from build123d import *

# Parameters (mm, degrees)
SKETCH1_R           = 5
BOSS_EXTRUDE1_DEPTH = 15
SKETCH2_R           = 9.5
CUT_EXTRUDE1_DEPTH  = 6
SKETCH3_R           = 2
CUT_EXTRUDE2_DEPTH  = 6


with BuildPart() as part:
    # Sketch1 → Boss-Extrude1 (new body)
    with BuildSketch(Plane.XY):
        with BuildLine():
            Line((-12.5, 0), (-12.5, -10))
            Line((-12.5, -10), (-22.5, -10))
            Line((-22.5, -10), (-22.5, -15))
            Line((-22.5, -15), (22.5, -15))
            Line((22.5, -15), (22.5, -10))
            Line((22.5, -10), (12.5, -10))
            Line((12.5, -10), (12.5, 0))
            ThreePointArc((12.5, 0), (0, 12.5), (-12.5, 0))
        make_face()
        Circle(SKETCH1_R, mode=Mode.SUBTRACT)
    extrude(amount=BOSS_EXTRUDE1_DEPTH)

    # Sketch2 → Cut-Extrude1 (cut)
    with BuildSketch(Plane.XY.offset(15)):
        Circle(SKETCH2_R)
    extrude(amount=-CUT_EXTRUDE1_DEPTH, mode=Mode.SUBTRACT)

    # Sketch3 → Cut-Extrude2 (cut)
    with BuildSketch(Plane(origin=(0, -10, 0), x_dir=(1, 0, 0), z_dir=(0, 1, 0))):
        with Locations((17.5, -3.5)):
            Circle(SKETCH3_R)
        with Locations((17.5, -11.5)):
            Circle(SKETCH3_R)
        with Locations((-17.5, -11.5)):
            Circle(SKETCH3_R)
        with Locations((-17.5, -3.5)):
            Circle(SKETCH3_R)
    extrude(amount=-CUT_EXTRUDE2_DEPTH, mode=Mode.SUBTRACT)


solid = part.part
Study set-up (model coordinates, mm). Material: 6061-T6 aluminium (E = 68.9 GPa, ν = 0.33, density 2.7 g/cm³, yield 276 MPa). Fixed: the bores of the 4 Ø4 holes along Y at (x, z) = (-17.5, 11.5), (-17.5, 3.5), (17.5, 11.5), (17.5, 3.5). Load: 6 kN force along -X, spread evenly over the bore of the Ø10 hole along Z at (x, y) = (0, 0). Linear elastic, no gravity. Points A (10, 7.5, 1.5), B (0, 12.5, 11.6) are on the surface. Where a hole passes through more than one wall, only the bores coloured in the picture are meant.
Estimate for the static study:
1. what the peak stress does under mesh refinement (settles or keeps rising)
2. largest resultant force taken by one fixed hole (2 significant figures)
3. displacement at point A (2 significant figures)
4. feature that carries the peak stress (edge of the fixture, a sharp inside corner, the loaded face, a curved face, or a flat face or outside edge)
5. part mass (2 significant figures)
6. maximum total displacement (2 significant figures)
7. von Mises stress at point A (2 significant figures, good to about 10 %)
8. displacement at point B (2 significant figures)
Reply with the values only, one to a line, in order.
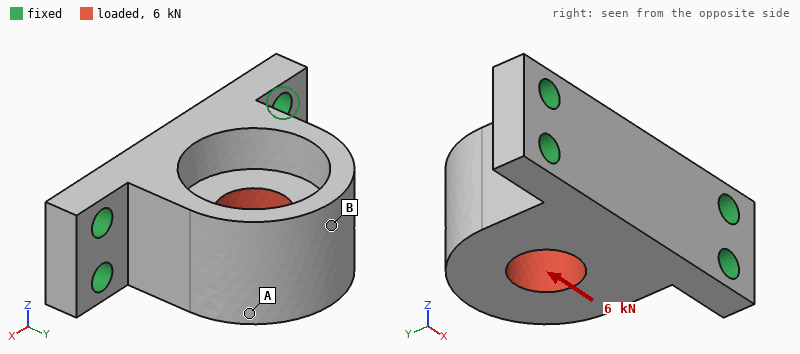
keeps rising
2.2 kN
48 µm
edge of the fixture
22 g
53 µm
33 MPa
51 µm
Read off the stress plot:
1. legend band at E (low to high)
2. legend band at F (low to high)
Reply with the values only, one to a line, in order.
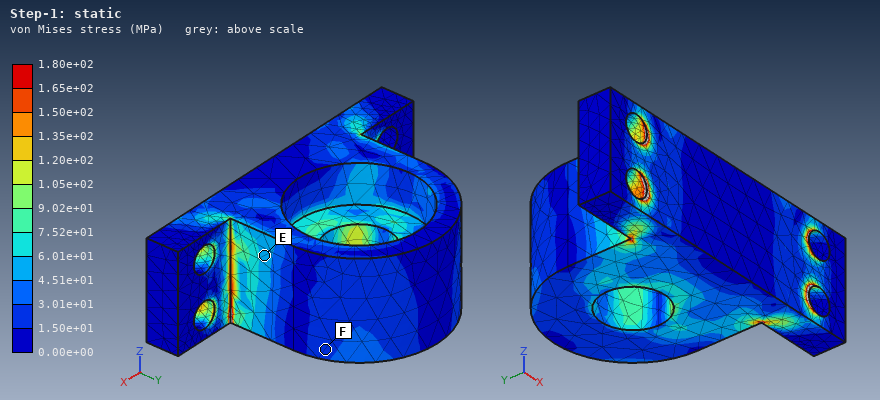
4.51e+01 to 6.01e+01 MPa
1.50e+01 to 3.01e+01 MPa
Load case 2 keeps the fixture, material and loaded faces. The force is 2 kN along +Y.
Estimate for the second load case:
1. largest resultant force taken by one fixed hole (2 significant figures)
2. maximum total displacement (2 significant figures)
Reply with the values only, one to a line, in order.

840 N
22 µm
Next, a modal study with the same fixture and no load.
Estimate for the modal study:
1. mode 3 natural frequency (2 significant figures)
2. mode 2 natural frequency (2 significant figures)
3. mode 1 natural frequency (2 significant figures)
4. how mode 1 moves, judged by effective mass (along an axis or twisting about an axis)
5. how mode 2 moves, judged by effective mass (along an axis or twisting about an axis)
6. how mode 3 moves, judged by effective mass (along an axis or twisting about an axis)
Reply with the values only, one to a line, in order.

20 kHz
16 kHz
7900 Hz
along Z
along X
along Y
